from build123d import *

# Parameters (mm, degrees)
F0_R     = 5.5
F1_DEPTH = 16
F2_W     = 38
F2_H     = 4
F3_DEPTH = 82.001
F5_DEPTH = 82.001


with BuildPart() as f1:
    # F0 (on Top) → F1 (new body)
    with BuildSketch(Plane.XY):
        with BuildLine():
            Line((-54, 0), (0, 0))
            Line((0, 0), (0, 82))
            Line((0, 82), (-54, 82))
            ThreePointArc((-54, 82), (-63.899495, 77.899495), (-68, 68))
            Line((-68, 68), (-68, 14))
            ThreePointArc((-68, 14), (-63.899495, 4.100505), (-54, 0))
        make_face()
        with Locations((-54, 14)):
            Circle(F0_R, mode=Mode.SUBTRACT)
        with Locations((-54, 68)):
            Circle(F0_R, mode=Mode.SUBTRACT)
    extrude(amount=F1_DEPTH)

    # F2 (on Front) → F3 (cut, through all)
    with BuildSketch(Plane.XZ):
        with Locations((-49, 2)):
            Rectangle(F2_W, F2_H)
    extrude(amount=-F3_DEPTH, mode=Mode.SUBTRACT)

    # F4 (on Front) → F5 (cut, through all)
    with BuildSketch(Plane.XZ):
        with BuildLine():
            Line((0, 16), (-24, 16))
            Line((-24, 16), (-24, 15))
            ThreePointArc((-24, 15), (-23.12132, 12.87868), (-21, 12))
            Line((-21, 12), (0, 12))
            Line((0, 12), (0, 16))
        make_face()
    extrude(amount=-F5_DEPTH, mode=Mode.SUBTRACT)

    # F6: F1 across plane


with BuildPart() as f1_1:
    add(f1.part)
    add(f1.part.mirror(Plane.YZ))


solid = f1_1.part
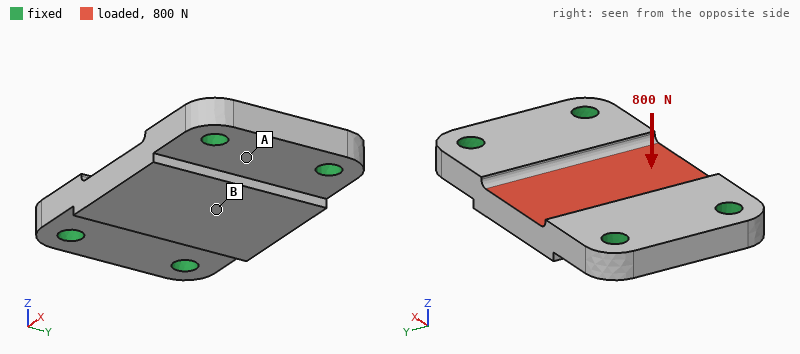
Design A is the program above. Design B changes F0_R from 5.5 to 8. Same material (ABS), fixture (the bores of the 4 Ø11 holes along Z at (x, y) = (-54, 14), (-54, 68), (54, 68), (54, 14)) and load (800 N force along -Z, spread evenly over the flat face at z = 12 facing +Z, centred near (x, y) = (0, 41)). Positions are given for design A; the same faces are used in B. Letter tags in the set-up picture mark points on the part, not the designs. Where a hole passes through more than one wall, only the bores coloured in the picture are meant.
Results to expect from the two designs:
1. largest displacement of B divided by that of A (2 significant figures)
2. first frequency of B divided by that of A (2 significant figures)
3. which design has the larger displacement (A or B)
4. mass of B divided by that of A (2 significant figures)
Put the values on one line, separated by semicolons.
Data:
0.81; 1.1; A; 0.96
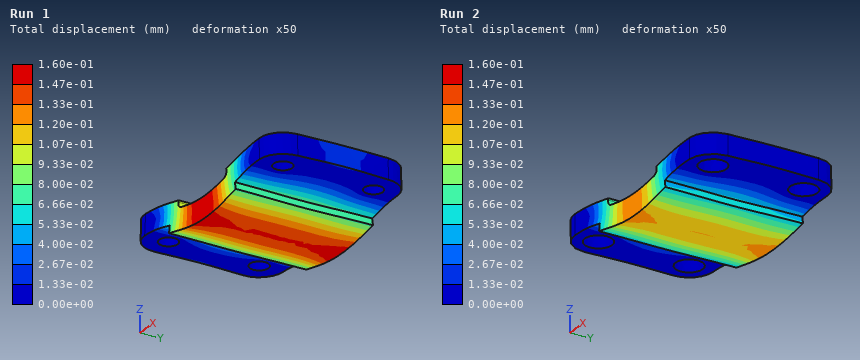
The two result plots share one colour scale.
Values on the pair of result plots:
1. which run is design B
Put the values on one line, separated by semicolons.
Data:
Run 2
